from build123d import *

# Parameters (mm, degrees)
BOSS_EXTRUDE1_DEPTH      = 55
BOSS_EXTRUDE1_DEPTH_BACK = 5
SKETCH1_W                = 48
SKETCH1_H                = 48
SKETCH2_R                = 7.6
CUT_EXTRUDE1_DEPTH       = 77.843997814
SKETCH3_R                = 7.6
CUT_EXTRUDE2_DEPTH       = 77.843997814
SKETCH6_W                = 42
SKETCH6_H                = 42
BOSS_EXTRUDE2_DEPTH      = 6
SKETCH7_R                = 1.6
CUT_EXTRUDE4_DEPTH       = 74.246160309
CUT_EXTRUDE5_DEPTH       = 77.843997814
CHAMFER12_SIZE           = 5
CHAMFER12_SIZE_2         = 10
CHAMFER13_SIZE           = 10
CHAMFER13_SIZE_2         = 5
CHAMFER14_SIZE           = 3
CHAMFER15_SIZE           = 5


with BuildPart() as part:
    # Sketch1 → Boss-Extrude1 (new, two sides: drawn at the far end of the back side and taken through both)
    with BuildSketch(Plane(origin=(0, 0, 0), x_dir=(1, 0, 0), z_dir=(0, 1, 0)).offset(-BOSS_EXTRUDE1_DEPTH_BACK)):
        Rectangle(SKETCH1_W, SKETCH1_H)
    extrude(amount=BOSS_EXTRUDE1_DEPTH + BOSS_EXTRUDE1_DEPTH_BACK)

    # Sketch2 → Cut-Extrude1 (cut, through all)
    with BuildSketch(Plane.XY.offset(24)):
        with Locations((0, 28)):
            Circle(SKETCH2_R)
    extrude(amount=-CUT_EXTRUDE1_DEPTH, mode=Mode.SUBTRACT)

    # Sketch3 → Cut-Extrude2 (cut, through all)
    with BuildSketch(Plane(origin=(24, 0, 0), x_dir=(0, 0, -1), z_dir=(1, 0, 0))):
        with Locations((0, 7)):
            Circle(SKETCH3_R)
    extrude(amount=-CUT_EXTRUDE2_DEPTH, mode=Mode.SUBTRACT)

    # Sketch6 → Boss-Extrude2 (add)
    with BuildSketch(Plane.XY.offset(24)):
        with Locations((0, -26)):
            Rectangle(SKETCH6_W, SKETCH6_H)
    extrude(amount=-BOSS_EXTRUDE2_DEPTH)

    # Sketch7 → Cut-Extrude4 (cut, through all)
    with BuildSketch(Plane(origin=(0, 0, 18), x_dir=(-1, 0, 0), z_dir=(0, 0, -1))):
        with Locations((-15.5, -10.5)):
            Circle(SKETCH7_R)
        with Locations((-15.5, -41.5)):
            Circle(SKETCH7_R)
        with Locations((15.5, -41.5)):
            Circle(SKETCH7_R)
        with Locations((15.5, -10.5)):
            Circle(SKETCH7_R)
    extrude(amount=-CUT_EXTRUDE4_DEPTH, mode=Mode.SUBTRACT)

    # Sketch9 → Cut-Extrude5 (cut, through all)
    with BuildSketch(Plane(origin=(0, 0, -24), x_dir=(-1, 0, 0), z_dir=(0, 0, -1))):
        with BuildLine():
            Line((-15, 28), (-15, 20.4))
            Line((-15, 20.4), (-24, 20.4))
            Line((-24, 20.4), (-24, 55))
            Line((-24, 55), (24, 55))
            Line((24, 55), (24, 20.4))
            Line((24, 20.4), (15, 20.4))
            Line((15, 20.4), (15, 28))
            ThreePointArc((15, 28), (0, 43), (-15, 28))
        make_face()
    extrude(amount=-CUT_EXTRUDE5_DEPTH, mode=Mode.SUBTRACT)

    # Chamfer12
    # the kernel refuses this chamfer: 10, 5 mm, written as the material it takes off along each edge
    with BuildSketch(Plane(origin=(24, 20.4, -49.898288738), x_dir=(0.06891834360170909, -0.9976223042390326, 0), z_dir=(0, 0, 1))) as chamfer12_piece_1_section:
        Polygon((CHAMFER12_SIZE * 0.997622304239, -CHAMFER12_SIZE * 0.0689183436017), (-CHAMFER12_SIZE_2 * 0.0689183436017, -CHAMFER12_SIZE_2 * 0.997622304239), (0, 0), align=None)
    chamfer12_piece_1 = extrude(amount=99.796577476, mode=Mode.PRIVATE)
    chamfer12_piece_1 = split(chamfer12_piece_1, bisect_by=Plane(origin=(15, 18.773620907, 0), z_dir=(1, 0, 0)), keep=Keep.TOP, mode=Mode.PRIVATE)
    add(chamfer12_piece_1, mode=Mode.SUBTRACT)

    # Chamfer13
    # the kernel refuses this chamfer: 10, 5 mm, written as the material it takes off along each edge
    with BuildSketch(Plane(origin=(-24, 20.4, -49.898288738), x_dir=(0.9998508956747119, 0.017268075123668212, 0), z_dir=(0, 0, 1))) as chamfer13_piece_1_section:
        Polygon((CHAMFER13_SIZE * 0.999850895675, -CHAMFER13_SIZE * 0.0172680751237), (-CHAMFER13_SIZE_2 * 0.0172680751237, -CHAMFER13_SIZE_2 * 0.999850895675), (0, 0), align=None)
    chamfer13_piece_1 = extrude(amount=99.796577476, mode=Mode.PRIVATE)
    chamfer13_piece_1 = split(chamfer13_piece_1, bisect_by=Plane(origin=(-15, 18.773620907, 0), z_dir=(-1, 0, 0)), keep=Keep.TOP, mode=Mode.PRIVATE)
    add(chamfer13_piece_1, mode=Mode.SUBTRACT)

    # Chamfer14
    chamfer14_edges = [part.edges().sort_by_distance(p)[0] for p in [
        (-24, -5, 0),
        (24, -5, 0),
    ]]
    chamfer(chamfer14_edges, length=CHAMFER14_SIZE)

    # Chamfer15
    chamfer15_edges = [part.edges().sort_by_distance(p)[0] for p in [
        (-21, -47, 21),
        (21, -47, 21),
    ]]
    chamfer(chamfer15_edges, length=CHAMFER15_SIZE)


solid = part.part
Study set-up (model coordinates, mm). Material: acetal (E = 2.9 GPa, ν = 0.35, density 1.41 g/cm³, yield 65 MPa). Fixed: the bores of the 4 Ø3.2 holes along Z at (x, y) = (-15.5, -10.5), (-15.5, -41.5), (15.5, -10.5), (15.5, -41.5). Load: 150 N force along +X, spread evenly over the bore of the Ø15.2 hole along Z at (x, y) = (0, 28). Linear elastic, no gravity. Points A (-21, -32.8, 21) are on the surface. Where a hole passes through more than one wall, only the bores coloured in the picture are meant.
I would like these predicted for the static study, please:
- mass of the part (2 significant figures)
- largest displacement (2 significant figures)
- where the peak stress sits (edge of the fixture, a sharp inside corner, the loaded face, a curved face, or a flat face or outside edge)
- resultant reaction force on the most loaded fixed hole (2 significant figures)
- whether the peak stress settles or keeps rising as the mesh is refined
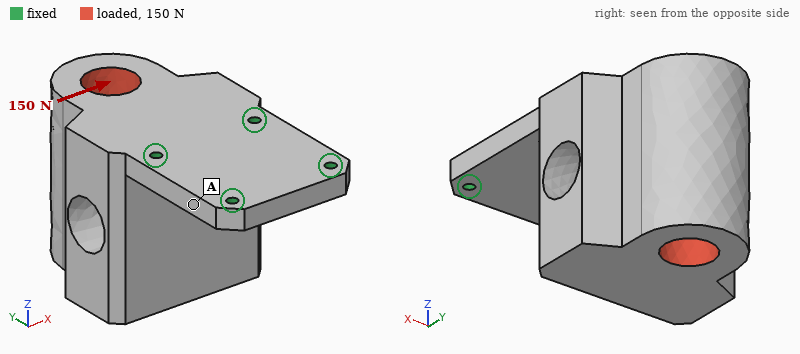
110 g
97 µm
edge of the fixture
210 N
keeps rising
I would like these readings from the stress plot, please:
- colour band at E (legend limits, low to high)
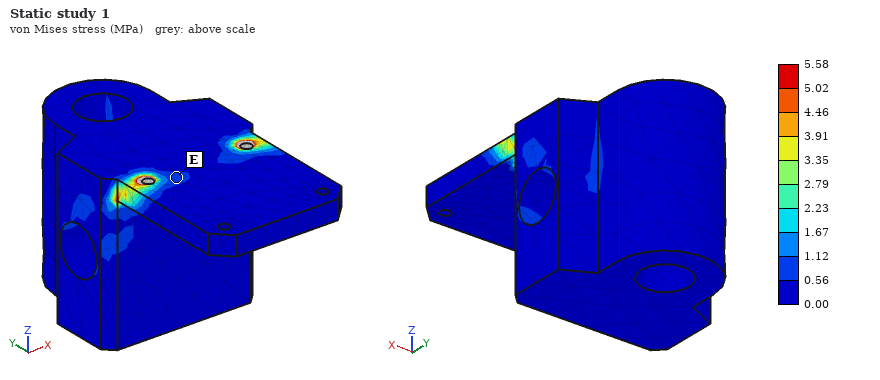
0.56 to 1.12 MPa
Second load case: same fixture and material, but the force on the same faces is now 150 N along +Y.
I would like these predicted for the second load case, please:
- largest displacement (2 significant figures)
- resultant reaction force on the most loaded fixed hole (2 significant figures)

0.93 mm
65 N
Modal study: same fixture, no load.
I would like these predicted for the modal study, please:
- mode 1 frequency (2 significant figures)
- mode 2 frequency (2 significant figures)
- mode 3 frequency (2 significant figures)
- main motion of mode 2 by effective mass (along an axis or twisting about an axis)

220 Hz
830 Hz
1600 Hz
along X
